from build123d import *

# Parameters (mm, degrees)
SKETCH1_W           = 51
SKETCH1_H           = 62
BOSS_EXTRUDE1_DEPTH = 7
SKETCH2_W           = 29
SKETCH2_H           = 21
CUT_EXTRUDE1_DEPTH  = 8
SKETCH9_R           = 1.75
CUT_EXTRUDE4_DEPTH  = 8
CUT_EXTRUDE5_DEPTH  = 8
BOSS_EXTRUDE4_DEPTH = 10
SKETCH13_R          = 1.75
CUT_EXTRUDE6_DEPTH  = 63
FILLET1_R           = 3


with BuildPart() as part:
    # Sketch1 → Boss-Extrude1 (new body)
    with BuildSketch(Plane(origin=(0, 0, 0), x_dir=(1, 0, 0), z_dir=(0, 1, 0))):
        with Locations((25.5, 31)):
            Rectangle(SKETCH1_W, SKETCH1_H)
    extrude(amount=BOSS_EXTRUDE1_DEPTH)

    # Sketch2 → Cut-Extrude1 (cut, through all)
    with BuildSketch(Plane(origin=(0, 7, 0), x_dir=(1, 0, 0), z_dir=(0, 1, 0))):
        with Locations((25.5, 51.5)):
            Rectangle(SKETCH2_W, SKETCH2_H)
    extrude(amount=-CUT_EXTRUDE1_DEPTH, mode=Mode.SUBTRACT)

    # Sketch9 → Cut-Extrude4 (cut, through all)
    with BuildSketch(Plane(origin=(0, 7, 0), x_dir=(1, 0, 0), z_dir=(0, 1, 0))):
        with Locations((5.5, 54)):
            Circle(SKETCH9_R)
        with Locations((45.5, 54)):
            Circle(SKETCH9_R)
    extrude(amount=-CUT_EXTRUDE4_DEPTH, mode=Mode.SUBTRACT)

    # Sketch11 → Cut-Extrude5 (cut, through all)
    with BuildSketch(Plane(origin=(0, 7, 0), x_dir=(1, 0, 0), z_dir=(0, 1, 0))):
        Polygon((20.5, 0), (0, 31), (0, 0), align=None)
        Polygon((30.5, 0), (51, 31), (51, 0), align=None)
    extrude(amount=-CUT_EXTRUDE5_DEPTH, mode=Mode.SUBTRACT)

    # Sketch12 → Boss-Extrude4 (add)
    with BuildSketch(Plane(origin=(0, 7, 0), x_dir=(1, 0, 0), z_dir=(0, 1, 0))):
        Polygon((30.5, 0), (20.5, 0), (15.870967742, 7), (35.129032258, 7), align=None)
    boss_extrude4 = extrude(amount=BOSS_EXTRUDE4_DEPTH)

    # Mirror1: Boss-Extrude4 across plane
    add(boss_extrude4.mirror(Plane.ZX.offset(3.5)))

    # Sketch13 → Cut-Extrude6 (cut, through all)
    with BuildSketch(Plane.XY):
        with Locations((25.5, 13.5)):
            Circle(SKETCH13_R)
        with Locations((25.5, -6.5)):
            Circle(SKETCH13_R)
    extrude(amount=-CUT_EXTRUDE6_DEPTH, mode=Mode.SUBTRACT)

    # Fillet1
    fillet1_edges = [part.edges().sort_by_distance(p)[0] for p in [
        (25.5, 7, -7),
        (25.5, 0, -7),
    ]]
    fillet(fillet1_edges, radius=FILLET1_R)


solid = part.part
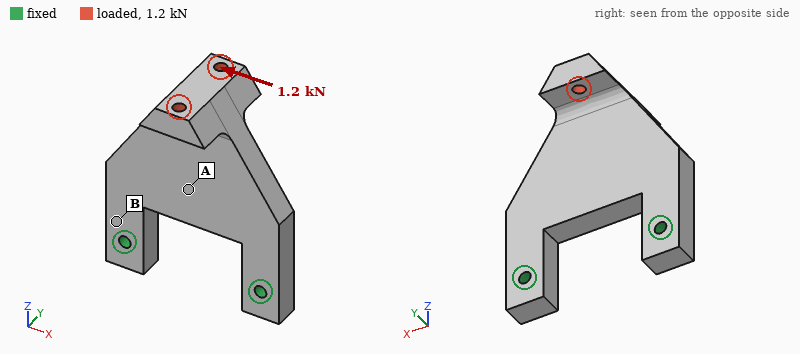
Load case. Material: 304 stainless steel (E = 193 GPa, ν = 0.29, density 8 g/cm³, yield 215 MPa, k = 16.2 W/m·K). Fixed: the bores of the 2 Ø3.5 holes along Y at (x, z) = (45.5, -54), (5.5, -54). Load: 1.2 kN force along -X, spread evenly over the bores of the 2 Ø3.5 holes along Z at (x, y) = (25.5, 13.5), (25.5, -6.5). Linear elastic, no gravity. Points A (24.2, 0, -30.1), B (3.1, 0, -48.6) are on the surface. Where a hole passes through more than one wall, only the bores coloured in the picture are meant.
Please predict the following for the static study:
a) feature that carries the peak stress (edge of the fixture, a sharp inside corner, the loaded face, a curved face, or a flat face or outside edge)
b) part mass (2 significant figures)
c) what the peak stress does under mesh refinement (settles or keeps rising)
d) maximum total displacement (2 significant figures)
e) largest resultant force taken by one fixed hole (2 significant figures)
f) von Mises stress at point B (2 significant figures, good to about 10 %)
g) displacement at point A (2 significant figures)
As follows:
edge of the fixture
120 g
keeps rising
13 µm
1.4 kN
25 MPa
6.2 µm
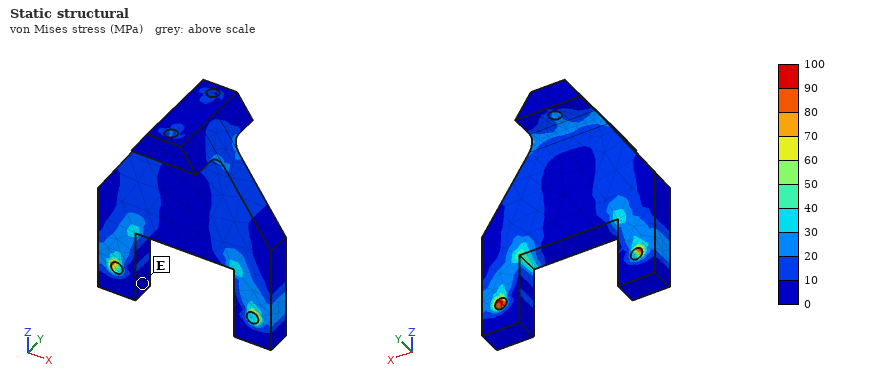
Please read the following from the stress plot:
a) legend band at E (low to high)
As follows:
0 to 10 MPa
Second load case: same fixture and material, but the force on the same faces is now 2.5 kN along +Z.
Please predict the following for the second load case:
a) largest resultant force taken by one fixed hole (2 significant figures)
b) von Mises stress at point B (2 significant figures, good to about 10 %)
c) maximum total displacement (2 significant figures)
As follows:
1.3 kN
15 MPa
11 µm
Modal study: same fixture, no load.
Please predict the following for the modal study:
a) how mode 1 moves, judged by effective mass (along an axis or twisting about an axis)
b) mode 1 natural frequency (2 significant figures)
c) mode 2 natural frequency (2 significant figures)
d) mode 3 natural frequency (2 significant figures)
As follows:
along Y
1400 Hz
6500 Hz
6700 Hz
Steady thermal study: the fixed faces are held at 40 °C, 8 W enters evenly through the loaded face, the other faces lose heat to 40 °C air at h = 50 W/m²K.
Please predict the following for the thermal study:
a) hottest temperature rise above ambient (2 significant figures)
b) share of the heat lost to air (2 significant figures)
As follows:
64 K
81 %
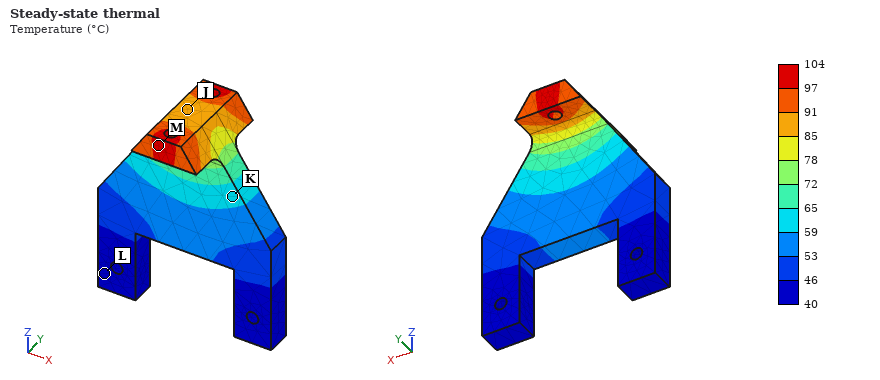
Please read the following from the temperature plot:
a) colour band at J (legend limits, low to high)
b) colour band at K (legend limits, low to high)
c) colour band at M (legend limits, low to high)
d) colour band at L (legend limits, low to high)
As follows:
85 to 91 °C
59 to 65 °C
97 to 104 °C
40 to 46 °C
